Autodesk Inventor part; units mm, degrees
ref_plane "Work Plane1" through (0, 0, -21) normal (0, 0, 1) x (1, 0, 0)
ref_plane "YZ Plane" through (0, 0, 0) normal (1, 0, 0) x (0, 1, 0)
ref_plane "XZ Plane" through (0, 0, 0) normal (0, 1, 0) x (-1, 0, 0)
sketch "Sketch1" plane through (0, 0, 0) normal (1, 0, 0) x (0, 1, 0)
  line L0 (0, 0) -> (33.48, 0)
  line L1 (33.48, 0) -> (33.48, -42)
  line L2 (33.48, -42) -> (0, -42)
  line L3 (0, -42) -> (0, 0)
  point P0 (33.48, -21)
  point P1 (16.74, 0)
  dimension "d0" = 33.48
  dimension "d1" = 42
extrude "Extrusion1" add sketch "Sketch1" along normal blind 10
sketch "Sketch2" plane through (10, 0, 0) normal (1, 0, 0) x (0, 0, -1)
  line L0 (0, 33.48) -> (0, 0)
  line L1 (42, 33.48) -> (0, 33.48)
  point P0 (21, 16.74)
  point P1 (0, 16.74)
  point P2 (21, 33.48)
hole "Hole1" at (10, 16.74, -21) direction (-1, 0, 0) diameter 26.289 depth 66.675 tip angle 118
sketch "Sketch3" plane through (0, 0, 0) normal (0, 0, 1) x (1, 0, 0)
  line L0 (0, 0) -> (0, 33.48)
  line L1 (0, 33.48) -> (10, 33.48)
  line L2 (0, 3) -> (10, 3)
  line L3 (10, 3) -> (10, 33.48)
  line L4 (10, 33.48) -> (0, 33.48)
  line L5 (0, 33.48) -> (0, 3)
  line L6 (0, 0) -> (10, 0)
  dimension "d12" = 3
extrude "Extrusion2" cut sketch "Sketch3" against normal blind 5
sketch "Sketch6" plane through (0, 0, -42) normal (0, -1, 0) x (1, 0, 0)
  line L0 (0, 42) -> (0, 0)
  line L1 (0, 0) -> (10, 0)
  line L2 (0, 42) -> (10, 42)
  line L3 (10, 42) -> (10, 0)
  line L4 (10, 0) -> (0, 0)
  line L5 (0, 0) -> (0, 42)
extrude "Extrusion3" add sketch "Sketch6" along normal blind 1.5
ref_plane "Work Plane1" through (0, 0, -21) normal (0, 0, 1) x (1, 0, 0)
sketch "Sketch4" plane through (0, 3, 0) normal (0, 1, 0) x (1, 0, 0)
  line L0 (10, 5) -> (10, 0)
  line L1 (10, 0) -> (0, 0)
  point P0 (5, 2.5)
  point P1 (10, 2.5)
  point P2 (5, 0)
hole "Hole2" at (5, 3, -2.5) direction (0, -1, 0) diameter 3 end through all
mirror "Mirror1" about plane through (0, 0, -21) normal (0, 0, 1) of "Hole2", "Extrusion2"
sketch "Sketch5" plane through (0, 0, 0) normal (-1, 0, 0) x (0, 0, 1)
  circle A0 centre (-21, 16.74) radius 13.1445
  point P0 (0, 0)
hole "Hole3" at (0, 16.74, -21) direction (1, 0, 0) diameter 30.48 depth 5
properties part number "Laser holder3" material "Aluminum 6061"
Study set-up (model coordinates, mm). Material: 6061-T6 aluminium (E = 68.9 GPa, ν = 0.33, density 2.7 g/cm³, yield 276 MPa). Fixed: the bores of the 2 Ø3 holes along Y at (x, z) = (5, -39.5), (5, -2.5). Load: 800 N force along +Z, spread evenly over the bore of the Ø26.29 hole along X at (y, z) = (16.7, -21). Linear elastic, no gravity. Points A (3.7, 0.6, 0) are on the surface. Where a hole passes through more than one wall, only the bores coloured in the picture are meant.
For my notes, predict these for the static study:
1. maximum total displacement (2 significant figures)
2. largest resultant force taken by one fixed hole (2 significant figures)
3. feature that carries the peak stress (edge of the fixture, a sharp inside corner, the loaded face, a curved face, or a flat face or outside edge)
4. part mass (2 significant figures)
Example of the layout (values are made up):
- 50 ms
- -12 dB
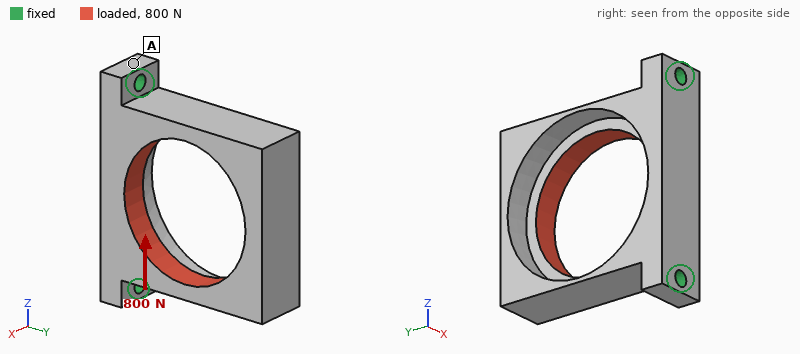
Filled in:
- 87 µm
- 540 N
- the loaded face
- 14 g
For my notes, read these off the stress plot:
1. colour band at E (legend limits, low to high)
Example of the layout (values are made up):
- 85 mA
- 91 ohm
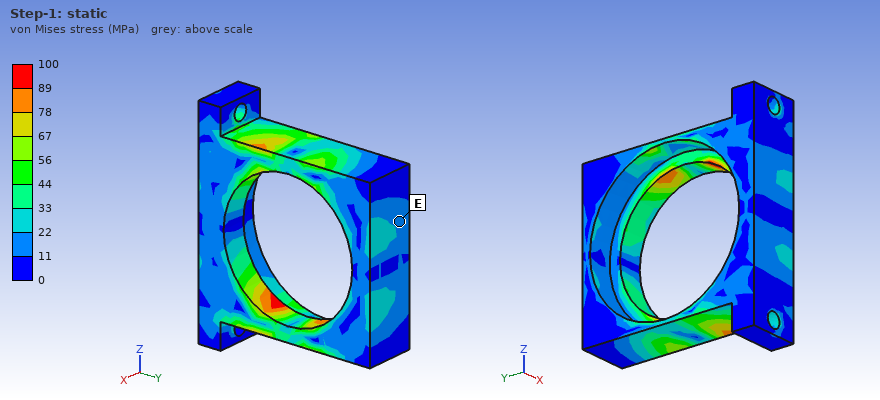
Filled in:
- 11 to 22 MPa
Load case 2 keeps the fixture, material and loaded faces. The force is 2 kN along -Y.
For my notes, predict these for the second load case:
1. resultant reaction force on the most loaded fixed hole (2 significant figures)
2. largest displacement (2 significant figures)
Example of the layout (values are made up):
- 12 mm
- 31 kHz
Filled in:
- 1.0 kN
- 87 µm
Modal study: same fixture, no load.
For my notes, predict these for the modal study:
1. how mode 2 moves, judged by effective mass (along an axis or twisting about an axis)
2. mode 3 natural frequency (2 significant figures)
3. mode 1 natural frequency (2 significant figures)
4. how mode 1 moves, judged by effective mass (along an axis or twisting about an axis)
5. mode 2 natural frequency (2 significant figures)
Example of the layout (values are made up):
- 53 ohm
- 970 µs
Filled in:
- along Z
- 6400 Hz
- 3000 Hz
- along X
- 4500 Hz
